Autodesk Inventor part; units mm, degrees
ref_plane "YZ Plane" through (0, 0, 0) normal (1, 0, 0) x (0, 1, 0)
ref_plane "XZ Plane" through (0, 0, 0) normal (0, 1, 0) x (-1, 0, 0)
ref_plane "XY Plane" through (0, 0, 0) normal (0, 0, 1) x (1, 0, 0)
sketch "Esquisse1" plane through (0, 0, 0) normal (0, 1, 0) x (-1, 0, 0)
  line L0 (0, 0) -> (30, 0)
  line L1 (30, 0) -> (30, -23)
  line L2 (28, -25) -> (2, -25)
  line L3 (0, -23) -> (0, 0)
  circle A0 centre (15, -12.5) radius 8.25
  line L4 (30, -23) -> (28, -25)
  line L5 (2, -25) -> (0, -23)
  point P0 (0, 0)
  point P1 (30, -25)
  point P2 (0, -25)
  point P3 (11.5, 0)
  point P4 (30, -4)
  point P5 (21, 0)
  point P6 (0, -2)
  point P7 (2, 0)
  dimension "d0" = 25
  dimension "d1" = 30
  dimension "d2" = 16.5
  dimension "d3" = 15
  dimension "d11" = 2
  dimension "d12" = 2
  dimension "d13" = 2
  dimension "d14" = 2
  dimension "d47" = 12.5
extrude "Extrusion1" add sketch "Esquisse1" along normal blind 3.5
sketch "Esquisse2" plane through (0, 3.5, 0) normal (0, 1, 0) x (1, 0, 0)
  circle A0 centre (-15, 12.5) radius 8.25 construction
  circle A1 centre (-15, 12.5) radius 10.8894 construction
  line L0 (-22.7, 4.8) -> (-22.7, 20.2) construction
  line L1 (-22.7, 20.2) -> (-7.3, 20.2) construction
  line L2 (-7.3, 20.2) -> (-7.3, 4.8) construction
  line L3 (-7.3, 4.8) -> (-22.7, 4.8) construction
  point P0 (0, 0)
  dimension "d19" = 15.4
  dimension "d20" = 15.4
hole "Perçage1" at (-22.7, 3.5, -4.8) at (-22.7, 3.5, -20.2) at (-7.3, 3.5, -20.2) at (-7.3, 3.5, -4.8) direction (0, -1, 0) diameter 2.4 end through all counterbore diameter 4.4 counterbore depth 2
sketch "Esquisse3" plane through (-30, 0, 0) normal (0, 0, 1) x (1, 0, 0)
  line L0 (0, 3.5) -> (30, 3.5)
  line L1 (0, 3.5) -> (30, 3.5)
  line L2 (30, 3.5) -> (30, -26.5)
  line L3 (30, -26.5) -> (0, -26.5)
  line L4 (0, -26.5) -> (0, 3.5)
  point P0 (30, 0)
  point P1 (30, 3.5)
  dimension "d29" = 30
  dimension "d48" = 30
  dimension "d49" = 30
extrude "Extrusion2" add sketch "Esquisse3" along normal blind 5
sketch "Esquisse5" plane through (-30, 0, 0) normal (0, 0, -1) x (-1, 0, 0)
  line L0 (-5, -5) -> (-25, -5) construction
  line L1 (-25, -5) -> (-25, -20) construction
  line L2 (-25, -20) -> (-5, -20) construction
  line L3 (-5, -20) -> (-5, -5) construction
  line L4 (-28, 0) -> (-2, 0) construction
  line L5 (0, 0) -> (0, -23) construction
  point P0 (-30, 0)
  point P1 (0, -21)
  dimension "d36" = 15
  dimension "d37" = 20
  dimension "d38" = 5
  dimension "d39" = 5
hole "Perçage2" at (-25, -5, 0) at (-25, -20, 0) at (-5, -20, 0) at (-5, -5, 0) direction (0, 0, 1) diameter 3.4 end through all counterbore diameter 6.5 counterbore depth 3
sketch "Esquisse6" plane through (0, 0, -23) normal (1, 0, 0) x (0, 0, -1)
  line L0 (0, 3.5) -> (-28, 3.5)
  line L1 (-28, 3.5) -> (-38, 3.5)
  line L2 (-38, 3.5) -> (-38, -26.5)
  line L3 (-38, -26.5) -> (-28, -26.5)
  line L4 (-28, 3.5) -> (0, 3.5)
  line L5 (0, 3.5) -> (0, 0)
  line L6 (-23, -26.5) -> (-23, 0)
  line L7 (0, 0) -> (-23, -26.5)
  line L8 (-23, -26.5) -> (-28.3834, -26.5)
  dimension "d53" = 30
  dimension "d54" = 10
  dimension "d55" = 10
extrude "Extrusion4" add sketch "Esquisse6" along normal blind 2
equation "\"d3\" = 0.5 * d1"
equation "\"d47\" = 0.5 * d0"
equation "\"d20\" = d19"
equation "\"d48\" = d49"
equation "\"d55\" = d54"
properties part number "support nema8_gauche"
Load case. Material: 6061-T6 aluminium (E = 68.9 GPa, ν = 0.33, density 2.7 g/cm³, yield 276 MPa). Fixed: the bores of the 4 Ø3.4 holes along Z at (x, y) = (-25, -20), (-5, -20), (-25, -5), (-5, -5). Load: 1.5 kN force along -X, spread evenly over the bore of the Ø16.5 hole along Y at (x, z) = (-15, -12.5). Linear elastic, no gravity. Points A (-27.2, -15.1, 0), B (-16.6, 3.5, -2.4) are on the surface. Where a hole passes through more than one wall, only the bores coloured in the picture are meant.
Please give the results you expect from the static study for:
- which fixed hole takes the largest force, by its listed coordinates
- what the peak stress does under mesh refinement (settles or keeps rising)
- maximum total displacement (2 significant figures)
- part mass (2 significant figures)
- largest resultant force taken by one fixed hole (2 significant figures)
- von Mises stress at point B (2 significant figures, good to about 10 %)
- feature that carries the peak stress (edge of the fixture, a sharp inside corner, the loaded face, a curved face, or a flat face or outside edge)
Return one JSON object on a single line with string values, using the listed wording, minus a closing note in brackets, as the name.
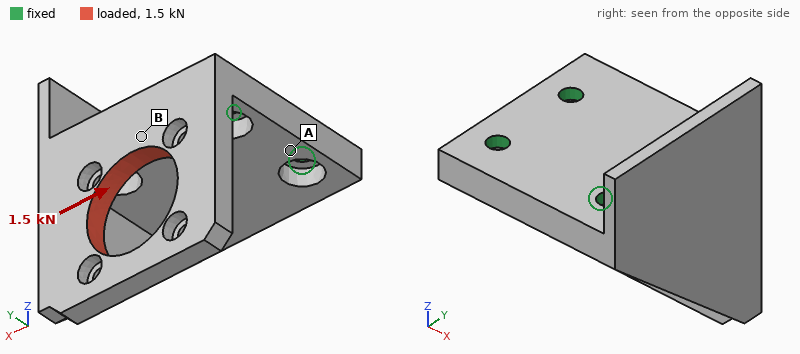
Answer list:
{"which fixed hole takes the largest force, by its listed coordinates": "(-25, -5)", "what the peak stress does under mesh refinement": "keeps rising", "maximum total displacement": "0.11 mm", "part mass": "20 g", "largest resultant force taken by one fixed hole": "1.5 kN", "von Mises stress at point B": "30 MPa", "feature that carries the peak stress": "edge of the fixture"}
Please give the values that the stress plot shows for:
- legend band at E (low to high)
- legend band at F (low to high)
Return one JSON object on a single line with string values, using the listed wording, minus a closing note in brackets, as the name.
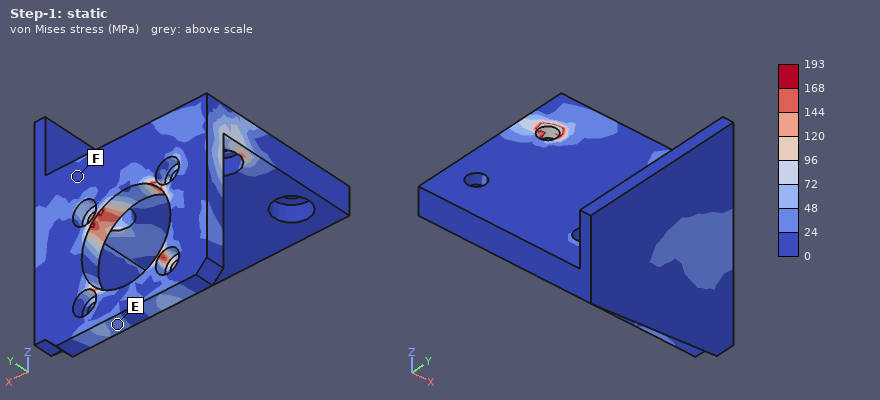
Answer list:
{"legend band at E": "24 to 48 MPa", "legend band at F": "0 to 24 MPa"}
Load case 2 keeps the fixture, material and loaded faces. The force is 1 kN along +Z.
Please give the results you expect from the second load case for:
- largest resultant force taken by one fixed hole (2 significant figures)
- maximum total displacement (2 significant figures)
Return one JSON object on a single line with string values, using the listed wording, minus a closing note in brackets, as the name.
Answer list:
{"largest resultant force taken by one fixed hole": "700 N", "maximum total displacement": "56 µm"}
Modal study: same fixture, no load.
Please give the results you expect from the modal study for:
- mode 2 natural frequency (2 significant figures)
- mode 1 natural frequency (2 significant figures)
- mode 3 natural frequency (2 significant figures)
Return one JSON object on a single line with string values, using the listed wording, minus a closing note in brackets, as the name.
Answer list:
{"mode 2 natural frequency": "8100 Hz", "mode 1 natural frequency": "4400 Hz", "mode 3 natural frequency": "11 kHz"}
